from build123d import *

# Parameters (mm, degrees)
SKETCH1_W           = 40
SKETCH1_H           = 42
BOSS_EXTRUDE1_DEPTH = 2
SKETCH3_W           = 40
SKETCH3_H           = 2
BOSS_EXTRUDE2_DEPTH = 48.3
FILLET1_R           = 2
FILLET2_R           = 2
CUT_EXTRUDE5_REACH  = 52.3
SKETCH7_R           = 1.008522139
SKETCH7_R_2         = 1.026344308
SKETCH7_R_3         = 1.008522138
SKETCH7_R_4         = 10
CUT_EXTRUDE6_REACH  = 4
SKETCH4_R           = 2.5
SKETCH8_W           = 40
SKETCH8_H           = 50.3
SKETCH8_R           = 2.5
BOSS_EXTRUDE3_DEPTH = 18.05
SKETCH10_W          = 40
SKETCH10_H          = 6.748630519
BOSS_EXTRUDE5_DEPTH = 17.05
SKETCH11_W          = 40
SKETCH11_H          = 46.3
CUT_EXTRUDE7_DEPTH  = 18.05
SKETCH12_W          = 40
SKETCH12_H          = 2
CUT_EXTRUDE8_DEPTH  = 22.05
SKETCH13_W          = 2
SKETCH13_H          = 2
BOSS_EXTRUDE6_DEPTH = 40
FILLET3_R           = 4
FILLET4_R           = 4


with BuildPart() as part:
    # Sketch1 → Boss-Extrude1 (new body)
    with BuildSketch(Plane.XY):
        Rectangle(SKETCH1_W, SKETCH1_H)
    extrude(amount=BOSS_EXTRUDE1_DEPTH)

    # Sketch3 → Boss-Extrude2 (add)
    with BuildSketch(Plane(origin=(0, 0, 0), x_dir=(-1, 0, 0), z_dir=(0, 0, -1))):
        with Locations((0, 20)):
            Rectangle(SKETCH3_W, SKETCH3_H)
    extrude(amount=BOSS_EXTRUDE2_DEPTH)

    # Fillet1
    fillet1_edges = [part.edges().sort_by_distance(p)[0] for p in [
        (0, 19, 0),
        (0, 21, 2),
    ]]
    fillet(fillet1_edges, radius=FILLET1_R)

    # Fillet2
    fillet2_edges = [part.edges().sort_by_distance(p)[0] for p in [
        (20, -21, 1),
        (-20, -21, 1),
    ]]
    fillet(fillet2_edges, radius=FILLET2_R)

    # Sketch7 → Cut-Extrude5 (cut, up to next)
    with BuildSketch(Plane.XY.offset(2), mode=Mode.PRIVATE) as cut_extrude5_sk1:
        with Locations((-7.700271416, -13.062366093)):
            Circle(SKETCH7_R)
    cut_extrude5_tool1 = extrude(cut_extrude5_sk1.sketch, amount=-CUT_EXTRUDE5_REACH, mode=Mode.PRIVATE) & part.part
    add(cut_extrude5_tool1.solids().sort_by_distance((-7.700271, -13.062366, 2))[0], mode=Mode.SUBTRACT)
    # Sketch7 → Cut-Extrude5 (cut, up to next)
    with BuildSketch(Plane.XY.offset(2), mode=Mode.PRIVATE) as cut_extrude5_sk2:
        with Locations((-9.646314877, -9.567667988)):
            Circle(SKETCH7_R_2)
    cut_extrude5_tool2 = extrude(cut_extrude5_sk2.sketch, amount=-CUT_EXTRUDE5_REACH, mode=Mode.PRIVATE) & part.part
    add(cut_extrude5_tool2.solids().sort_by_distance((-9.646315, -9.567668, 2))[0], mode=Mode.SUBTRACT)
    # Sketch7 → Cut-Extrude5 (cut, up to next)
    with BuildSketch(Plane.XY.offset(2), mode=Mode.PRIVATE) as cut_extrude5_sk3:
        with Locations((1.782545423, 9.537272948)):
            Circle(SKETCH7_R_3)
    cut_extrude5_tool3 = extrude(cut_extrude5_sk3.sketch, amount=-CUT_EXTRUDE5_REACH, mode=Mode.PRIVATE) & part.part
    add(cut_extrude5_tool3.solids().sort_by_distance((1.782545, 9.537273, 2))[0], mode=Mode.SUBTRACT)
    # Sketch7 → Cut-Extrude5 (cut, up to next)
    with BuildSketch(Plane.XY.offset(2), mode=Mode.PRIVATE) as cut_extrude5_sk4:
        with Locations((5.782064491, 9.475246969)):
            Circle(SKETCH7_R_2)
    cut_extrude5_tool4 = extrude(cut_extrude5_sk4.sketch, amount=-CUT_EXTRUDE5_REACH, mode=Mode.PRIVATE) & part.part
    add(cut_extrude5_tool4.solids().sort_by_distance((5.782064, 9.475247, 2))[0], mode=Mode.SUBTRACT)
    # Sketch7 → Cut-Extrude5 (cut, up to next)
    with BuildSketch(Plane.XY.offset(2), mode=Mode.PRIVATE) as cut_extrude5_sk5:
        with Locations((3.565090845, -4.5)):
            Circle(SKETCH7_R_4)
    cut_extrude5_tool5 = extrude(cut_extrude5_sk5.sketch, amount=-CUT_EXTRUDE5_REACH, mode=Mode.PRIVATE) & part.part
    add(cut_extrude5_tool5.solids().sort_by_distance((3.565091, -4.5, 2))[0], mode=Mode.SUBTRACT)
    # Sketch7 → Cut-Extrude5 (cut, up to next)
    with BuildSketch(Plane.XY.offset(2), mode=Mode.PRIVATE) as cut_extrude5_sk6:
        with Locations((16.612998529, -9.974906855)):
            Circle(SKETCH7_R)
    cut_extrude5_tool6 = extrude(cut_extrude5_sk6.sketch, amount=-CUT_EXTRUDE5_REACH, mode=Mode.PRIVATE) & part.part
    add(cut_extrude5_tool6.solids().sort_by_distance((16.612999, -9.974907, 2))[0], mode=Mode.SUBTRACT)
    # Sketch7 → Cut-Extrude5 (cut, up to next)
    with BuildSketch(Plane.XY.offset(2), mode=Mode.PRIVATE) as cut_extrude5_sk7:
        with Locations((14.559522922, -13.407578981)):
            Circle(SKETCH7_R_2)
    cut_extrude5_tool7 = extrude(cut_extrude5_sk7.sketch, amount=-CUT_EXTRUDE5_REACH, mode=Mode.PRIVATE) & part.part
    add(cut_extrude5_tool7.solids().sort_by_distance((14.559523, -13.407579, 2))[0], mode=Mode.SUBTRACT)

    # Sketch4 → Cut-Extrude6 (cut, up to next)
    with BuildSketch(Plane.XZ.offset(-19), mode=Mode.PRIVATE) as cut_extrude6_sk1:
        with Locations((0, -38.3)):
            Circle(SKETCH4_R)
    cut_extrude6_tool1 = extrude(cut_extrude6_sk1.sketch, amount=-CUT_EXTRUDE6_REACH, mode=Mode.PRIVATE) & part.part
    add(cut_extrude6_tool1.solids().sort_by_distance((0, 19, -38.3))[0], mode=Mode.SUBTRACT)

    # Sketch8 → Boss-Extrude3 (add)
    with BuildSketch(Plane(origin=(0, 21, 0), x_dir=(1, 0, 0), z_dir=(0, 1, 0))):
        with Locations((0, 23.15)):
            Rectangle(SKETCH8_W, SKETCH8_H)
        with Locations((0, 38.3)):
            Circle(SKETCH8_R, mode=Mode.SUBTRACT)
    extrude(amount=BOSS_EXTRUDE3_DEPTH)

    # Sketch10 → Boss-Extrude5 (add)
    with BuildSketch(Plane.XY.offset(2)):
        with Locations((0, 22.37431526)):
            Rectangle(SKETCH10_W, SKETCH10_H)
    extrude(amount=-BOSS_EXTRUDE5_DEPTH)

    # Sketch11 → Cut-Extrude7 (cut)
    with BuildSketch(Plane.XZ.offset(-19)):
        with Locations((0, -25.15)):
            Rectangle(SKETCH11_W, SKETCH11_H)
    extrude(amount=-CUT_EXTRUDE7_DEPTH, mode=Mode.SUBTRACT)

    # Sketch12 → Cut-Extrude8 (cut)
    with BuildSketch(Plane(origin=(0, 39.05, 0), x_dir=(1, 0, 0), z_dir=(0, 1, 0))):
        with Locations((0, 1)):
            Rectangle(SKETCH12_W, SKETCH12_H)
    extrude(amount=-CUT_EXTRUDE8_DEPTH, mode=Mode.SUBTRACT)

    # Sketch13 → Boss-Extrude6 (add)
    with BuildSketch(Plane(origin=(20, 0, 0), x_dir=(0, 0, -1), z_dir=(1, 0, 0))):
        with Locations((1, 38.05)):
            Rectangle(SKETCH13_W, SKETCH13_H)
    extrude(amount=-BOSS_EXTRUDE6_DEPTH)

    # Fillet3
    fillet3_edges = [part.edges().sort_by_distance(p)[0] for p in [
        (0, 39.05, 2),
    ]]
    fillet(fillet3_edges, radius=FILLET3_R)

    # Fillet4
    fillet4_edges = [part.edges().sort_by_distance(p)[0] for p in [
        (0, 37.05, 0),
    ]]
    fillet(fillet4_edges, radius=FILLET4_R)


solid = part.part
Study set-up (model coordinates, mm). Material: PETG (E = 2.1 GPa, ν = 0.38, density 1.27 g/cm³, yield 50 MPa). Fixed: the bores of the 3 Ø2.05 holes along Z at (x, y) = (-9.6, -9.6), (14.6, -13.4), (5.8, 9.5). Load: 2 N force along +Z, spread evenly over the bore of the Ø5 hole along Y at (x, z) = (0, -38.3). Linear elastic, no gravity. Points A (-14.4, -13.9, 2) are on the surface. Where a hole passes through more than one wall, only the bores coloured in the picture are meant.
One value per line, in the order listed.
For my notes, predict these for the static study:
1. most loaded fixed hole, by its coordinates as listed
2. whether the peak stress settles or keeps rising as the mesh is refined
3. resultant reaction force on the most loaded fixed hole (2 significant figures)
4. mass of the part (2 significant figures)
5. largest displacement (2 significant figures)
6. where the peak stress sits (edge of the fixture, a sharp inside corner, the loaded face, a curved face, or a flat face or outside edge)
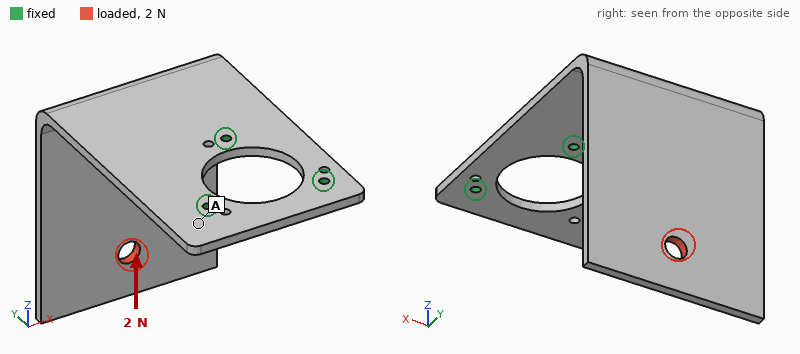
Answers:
(5.8, 9.5)
keeps rising
3.1 N
10 g
0.98 mm
edge of the fixture
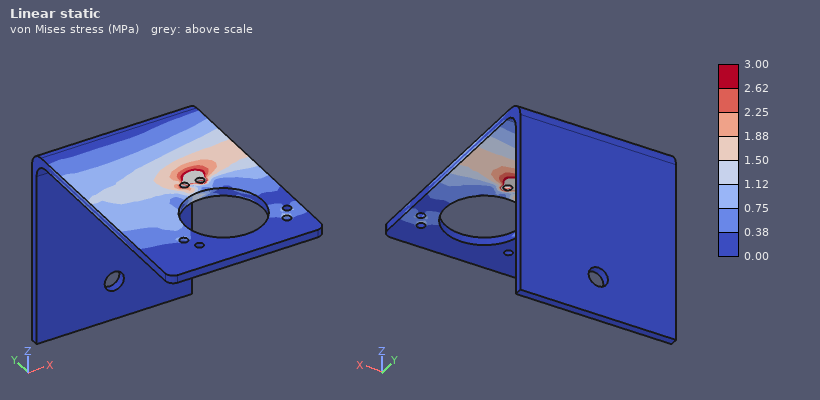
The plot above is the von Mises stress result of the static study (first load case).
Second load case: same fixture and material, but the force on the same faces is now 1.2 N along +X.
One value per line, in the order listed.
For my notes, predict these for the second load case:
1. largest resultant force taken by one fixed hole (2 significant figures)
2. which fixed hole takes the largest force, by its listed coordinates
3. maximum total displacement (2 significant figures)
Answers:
1.7 N
(5.8, 9.5)
0.90 mm
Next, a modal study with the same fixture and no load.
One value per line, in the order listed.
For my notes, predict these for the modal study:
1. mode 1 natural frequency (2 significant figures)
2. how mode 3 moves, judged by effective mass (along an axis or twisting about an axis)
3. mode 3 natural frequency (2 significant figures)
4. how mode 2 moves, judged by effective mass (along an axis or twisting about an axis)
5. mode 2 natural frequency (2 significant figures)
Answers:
87 Hz
along Z
270 Hz
along X
130 Hz
